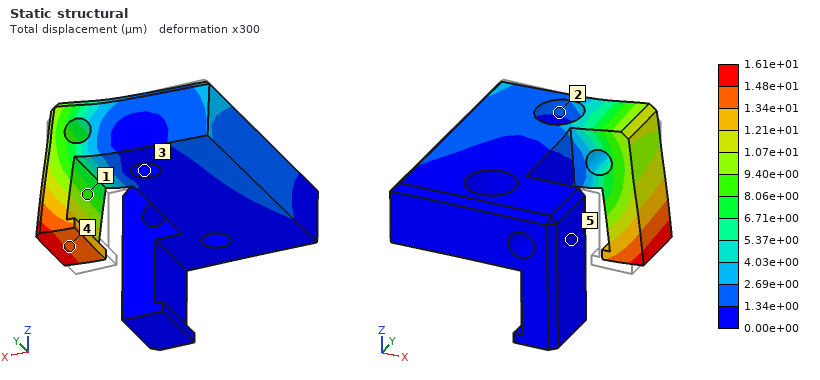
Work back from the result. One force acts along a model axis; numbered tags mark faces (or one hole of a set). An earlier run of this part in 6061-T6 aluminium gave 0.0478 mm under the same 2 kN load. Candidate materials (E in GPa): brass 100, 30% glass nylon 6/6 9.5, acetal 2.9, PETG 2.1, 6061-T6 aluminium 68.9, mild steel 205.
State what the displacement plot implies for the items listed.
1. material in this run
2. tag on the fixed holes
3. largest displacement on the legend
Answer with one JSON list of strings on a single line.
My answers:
["mild steel", "3", "1.61e+01 µm"]
